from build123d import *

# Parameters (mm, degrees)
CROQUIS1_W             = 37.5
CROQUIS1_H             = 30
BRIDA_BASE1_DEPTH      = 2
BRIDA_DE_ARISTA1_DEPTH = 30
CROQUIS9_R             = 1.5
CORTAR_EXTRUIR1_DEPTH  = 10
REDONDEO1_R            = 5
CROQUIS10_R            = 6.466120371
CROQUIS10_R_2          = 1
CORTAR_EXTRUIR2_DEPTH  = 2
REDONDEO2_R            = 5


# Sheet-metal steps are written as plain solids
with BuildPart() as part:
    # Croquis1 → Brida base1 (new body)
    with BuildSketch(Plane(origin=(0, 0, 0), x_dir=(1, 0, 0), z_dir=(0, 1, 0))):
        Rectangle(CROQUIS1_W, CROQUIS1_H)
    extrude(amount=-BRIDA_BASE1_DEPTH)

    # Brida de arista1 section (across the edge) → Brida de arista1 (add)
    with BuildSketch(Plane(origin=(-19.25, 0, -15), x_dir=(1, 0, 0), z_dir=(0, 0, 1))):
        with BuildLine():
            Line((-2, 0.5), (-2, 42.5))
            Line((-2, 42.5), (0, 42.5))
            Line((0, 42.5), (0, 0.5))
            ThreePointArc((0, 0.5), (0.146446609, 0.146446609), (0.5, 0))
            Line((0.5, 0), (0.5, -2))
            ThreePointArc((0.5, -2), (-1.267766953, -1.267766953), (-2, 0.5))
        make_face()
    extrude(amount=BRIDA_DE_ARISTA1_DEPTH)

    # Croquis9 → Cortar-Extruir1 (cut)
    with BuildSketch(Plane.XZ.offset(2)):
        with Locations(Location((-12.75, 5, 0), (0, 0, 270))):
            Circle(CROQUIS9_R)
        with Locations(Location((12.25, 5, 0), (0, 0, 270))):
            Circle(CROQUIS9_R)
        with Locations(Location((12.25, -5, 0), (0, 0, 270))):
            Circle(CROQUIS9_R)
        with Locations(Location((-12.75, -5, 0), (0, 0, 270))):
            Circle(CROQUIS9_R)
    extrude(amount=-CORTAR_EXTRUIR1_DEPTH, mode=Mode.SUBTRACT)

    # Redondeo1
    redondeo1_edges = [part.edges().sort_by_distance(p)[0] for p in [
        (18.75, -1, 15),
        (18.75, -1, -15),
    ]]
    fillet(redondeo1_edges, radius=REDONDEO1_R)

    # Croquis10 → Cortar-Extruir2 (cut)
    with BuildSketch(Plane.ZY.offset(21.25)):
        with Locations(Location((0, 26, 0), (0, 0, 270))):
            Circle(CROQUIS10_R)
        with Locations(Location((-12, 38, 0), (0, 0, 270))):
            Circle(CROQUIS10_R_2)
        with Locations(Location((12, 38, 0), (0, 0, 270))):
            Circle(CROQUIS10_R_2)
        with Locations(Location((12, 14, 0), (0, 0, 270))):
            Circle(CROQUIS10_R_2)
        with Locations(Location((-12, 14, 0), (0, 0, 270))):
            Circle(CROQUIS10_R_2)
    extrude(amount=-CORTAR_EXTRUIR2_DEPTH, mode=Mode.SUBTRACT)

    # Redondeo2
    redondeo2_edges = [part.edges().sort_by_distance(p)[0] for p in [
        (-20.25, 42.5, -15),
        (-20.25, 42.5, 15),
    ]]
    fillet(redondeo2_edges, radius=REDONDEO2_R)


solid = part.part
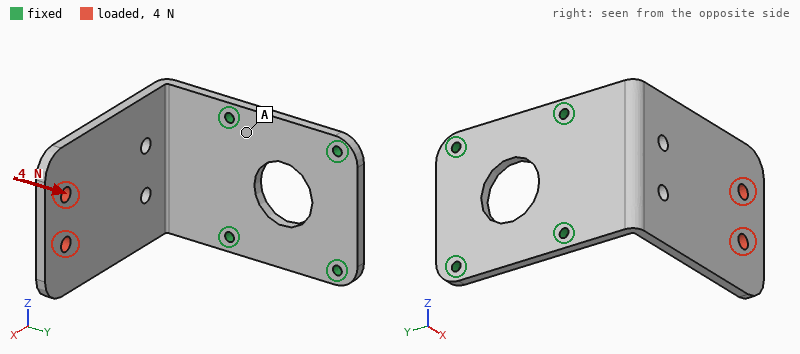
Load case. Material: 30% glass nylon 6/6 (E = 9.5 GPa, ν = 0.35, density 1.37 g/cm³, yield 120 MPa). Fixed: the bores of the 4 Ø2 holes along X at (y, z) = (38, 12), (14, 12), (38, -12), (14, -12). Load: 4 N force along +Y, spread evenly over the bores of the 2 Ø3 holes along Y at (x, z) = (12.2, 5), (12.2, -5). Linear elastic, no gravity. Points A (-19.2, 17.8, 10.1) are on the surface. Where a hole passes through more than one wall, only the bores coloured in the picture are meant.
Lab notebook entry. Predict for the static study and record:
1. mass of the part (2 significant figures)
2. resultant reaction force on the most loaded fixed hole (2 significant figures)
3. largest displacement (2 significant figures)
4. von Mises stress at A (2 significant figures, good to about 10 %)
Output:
6.2 g
2.1 N
0.71 mm
1.1 MPa
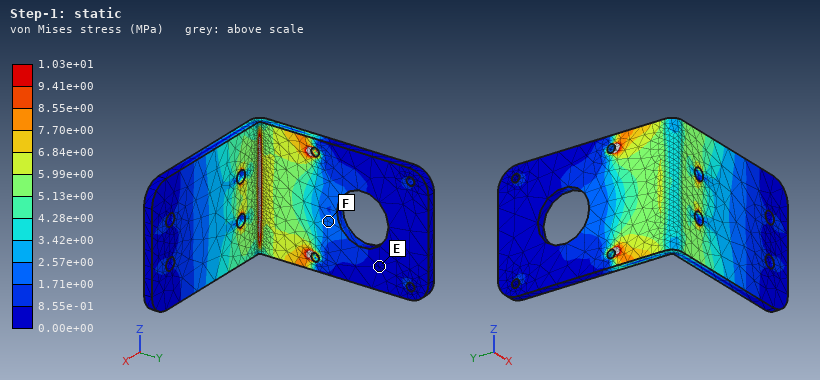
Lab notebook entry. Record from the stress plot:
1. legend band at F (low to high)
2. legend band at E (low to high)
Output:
1.71e+00 to 2.57e+00 MPa
0.00e+00 to 8.55e-01 MPa
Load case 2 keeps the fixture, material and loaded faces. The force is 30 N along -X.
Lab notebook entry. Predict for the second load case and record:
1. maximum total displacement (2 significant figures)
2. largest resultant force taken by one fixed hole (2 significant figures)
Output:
0.80 mm
17 N
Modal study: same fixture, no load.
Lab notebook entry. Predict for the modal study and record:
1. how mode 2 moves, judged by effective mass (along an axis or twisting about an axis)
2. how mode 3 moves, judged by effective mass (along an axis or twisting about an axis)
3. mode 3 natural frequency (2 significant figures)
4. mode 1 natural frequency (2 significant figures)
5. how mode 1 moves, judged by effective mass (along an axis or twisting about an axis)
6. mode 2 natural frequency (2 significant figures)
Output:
along Z
along X
1400 Hz
350 Hz
along Y
800 Hz
